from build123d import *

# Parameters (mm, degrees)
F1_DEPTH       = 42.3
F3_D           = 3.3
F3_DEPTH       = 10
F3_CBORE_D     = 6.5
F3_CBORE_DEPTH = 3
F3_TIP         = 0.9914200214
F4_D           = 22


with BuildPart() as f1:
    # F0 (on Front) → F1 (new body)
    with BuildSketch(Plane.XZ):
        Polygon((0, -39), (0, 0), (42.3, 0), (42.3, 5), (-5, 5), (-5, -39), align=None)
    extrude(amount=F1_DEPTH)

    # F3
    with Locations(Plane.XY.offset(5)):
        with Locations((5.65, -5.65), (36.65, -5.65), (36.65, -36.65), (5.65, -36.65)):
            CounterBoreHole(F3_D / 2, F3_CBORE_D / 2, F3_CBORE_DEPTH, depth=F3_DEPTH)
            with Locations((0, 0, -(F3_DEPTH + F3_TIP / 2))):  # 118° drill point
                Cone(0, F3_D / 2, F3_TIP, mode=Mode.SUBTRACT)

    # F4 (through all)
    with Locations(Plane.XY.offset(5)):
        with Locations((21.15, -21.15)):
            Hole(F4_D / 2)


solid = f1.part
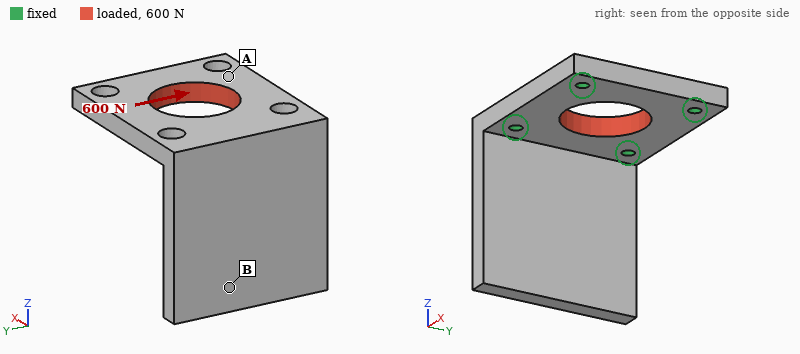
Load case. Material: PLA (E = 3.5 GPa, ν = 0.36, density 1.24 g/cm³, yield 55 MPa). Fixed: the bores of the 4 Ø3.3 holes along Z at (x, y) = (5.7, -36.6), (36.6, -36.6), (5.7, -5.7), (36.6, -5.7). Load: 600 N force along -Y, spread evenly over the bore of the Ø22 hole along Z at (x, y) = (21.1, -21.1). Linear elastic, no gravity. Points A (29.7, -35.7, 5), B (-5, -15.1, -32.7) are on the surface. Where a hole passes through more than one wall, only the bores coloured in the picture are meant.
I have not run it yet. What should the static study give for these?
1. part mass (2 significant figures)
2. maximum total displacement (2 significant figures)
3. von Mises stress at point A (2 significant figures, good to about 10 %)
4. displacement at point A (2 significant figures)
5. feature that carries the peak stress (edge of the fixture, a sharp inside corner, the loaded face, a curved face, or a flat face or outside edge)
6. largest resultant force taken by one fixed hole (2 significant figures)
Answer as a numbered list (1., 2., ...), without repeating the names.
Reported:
1. 20 g
2. 32 µm
3. 2.8 MPa
4. 20 µm
5. edge of the fixture
6. 160 N
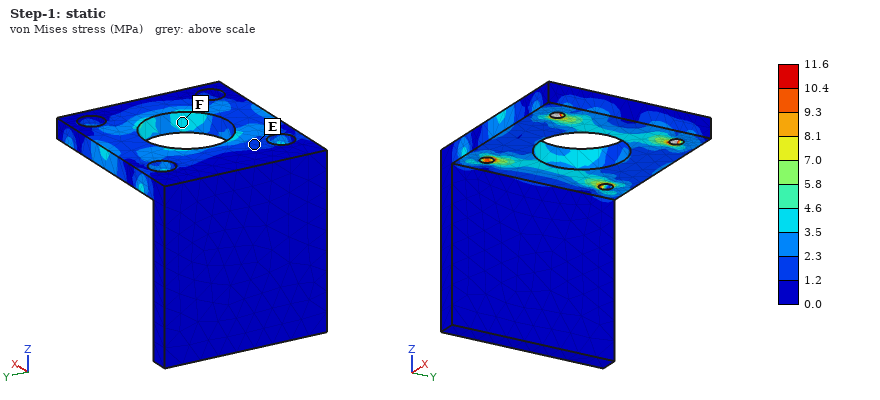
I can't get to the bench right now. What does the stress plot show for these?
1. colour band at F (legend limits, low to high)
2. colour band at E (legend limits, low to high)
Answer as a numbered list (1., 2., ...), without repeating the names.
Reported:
1. 3.5 to 4.6 MPa
2. 1.2 to 2.3 MPa
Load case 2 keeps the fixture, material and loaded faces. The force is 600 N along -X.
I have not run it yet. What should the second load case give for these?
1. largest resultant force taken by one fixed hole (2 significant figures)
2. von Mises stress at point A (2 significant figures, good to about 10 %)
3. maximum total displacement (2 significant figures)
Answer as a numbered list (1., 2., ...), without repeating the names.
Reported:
1. 150 N
2. 1.5 MPa
3. 67 µm
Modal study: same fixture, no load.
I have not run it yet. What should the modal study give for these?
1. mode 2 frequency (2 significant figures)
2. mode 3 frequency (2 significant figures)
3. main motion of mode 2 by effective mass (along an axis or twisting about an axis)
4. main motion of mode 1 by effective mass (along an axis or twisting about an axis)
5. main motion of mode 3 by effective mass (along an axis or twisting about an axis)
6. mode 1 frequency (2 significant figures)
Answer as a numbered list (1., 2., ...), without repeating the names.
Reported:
1. 1400 Hz
2. 1900 Hz
3. along Y
4. along X
5. along Y
6. 510 Hz
